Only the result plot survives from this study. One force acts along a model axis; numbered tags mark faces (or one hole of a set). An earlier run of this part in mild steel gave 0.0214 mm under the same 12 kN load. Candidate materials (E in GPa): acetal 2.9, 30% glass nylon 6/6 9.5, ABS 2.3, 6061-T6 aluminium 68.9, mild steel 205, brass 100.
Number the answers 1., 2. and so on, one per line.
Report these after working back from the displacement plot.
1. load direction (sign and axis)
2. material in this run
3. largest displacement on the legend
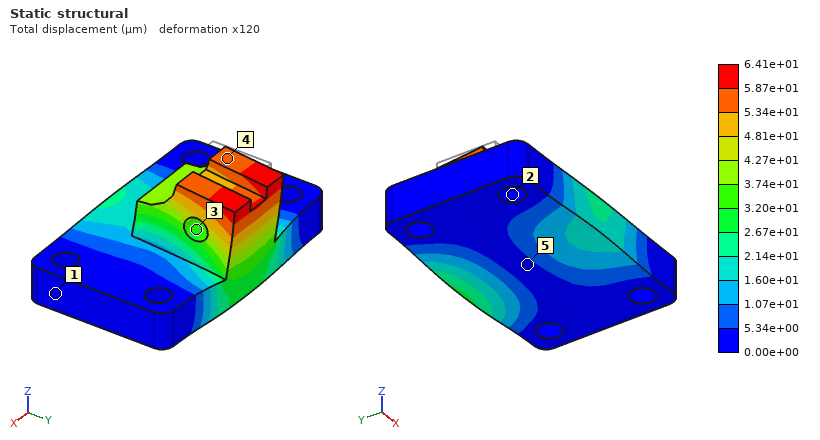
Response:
1. +Y
2. 6061-T6 aluminium
3. 6.41e+01 µm
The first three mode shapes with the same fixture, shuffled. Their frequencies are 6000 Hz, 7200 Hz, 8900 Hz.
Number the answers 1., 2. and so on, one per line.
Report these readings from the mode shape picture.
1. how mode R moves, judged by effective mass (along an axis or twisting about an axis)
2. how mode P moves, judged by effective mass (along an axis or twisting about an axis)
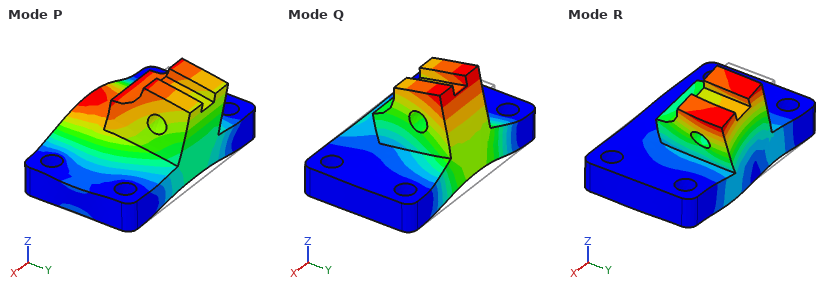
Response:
1. along X
2. along Z
